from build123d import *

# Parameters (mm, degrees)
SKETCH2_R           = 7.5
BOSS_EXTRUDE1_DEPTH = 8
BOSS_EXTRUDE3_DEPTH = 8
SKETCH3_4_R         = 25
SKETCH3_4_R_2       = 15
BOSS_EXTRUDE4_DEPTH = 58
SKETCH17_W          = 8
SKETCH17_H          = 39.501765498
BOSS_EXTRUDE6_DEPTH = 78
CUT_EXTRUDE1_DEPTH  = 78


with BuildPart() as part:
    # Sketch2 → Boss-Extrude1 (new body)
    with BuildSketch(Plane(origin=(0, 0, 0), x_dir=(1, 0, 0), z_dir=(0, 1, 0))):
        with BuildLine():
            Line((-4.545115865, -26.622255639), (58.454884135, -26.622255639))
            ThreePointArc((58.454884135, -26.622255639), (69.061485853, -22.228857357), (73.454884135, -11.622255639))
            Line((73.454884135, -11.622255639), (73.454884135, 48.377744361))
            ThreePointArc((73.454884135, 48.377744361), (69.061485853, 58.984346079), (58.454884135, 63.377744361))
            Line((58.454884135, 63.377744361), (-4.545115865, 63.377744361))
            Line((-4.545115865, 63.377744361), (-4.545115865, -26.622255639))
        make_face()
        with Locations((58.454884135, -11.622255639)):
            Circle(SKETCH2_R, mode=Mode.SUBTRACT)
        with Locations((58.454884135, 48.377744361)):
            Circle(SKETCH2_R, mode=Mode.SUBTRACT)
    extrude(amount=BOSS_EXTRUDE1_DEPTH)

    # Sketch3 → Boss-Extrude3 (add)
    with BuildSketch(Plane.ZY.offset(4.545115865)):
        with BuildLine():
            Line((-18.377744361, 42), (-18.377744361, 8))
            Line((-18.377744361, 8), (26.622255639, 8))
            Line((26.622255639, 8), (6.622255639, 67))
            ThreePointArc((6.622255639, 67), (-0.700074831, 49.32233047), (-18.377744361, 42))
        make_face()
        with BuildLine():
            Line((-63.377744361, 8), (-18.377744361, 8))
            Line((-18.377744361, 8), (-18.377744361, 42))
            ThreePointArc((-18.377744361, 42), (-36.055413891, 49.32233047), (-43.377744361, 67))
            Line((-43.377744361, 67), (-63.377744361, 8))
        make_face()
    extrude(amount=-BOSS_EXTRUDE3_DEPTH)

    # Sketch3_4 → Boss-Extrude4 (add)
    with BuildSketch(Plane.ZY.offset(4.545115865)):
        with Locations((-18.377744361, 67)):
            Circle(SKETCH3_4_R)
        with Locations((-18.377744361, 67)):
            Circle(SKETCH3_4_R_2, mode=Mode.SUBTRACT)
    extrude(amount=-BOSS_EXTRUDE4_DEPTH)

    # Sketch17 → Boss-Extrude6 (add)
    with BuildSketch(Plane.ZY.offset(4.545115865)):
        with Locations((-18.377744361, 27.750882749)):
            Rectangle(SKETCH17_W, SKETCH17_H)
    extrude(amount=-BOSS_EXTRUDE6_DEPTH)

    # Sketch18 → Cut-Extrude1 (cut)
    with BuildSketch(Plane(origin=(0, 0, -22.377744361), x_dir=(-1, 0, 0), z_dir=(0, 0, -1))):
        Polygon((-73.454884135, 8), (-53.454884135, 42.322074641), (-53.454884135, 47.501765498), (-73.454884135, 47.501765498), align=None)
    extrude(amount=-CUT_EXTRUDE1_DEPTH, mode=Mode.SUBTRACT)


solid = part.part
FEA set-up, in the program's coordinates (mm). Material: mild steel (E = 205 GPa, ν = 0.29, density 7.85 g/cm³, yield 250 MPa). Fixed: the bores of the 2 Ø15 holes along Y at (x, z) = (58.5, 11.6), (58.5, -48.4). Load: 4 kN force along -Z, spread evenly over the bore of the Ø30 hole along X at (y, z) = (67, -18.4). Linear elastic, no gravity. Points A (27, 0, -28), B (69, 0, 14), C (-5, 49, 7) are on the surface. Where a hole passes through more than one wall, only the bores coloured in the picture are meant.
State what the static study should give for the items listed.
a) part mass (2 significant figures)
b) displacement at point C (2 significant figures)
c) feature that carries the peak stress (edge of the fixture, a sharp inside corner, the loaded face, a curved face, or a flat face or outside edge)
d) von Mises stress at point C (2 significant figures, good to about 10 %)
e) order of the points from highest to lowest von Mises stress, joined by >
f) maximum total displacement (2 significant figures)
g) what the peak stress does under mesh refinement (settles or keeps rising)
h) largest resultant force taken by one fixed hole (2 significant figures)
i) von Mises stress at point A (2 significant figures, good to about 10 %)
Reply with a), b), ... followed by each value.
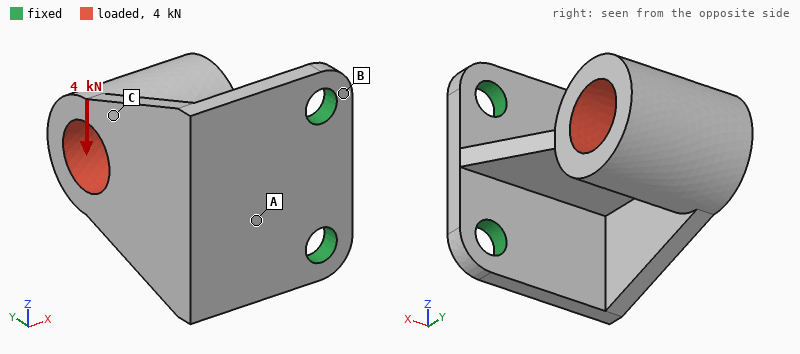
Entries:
a) 1.3 kg
b) 0.17 mm
c) edge of the fixture
d) 31 MPa
e) A > C > B
f) 0.30 mm
g) keeps rising
h) 5.5 kN
i) 85 MPa
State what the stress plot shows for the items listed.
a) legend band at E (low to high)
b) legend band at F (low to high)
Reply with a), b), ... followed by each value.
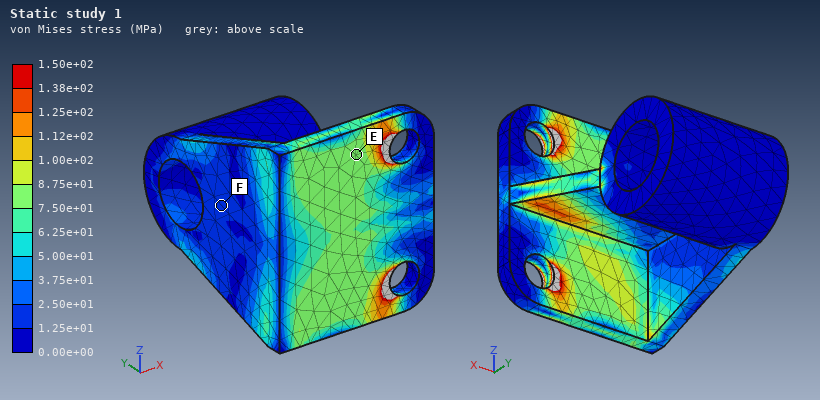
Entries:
a) 7.50e+01 to 8.75e+01 MPa
b) 1.25e+01 to 2.50e+01 MPa
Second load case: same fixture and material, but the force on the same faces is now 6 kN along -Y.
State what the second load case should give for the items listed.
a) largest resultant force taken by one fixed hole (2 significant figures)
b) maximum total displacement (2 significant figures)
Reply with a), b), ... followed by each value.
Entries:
a) 3.0 kN
b) 0.23 mm
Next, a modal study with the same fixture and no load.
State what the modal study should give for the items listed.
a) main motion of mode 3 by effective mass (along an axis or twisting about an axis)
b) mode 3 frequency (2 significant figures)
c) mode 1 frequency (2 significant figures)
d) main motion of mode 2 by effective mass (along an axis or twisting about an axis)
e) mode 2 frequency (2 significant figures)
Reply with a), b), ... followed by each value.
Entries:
a) twisting about Y
b) 2900 Hz
c) 690 Hz
d) along Z
e) 800 Hz
